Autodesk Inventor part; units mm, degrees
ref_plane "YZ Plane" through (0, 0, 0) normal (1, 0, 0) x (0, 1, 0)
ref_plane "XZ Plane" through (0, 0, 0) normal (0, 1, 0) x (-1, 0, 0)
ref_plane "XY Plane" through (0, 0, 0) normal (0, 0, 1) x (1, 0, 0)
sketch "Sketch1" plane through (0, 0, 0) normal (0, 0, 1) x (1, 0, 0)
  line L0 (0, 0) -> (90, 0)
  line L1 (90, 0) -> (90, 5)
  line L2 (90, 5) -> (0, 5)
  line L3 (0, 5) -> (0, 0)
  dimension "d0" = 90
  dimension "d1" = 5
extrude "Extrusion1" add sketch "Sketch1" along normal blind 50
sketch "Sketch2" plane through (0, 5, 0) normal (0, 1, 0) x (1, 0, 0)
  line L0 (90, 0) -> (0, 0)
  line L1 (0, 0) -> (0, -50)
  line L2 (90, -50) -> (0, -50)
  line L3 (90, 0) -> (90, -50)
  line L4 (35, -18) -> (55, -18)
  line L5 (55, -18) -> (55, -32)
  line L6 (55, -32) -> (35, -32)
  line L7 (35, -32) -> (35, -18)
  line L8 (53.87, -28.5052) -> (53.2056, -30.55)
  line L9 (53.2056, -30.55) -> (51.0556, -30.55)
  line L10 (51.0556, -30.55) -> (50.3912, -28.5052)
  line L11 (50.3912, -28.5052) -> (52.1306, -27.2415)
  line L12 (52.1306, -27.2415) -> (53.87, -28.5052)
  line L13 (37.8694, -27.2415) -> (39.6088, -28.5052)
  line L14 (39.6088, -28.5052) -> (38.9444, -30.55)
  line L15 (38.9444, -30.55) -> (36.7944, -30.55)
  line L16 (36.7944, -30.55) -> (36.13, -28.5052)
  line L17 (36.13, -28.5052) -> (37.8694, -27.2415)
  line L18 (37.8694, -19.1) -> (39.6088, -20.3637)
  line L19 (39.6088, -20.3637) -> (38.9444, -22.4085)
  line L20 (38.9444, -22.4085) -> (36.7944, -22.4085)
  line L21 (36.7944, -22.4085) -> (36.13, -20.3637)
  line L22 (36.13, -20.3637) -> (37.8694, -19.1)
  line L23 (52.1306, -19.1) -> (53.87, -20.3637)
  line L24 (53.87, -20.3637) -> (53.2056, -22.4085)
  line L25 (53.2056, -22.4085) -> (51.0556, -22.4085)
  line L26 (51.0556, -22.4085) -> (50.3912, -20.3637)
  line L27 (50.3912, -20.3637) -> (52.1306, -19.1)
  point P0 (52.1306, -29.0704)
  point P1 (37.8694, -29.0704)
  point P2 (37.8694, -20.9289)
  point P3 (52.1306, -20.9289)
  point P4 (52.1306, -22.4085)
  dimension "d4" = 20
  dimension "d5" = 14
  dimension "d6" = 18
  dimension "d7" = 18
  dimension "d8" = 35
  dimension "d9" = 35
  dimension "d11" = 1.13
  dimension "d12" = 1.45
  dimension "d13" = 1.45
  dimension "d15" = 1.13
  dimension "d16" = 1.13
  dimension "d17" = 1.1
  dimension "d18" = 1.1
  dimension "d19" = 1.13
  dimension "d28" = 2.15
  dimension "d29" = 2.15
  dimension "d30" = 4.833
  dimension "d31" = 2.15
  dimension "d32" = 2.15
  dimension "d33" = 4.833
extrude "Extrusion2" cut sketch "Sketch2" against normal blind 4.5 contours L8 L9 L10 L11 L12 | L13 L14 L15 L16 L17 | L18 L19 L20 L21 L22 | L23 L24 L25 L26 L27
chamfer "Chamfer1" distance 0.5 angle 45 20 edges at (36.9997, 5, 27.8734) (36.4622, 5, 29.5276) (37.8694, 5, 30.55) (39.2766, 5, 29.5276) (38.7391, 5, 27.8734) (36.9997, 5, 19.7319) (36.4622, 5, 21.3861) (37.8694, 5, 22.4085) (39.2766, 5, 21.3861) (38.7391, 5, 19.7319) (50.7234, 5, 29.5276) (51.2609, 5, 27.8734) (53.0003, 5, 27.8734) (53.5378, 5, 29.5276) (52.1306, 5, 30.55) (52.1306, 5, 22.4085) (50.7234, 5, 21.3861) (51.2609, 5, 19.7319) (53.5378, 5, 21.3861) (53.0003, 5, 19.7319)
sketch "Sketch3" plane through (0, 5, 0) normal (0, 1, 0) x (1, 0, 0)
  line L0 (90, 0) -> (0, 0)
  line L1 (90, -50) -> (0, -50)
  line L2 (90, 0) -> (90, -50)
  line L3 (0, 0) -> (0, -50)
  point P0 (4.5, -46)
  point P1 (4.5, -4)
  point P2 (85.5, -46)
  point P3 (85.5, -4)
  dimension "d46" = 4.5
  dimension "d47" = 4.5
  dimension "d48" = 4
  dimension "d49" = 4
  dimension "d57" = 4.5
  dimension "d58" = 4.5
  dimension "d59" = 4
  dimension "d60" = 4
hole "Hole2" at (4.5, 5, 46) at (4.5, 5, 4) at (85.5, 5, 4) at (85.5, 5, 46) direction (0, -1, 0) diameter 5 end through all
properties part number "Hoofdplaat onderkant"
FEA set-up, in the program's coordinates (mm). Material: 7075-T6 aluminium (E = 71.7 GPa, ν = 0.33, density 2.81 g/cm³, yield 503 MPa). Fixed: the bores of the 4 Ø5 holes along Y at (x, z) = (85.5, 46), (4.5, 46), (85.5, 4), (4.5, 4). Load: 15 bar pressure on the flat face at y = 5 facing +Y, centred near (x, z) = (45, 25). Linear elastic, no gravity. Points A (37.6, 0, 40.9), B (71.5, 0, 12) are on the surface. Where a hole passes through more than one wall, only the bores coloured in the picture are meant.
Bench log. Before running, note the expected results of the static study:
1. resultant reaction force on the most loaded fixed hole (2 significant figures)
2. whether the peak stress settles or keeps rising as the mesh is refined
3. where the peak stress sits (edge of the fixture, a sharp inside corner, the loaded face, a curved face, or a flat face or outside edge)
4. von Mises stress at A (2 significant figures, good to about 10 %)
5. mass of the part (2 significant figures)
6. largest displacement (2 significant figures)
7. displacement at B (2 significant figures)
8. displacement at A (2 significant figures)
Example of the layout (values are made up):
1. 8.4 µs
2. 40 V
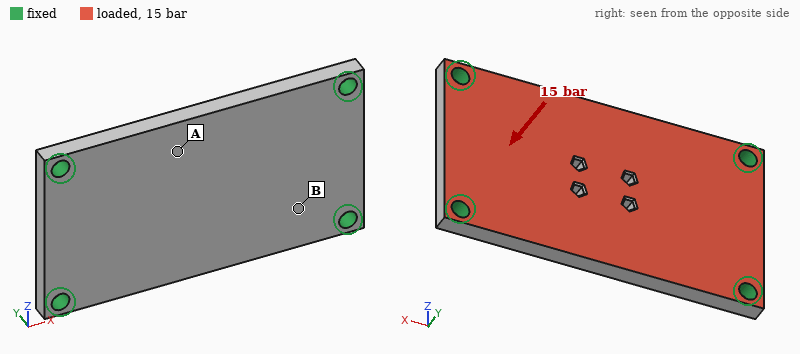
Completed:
1. 1.6 kN
2. keeps rising
3. edge of the fixture
4. 97 MPa
5. 62 g
6. 0.28 mm
7. 0.12 mm
8. 0.26 mm
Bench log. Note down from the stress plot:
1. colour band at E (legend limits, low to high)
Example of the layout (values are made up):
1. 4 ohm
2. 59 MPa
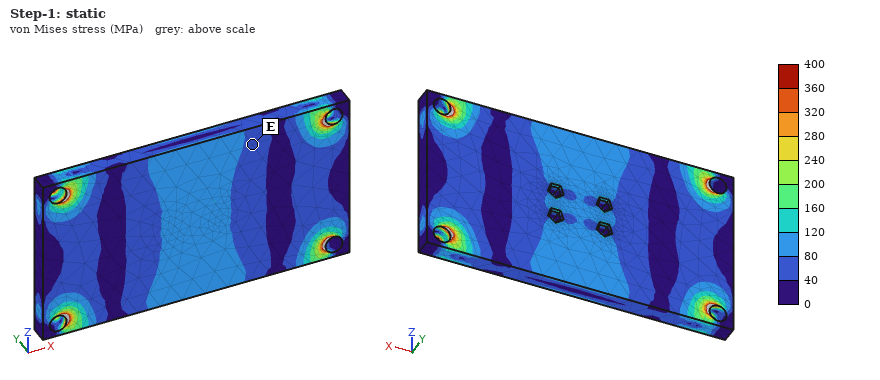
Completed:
1. 40 to 80 MPa
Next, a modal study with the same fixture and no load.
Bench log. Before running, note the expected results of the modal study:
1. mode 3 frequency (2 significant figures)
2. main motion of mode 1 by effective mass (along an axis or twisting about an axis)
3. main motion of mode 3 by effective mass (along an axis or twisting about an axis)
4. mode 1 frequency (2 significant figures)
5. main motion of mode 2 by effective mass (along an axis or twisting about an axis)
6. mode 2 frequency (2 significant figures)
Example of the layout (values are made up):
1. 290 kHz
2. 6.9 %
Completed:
1. 9300 Hz
2. along Y
3. twisting about Z
4. 3500 Hz
5. twisting about X
6. 5800 Hz
